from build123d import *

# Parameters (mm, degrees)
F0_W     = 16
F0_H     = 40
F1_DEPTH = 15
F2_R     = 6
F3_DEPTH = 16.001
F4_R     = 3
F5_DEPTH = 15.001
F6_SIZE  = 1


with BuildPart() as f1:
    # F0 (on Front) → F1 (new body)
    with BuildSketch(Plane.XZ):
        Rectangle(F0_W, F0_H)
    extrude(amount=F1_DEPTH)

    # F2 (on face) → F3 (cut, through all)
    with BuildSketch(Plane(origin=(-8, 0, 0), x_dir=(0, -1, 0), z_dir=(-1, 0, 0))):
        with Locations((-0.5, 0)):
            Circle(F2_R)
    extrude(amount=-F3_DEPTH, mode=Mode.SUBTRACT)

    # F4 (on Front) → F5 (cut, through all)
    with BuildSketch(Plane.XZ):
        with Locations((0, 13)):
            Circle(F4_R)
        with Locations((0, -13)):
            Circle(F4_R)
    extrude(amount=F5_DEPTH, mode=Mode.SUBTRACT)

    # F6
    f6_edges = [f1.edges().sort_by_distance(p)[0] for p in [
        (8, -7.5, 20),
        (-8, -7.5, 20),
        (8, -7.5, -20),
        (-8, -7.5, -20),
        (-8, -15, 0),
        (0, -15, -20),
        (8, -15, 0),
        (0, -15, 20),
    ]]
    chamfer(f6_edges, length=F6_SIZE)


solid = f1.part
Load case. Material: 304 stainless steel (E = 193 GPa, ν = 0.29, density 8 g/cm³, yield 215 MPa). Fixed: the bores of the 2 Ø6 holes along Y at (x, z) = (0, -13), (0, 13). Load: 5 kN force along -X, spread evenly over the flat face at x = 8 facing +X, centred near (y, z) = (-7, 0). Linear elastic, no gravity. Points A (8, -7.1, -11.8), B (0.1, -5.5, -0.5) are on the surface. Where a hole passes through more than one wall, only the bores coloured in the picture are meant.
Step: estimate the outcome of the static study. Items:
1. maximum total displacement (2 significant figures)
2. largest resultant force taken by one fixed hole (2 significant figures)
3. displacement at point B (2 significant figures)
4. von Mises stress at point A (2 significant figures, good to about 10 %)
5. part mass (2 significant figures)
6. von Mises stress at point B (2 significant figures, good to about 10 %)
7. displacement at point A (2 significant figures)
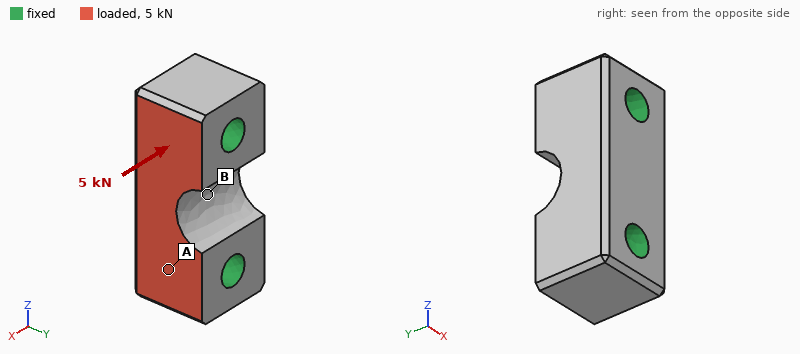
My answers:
0.96 µm
2.5 kN
0.68 µm
14 MPa
63 g
5.3 MPa
0.39 µm
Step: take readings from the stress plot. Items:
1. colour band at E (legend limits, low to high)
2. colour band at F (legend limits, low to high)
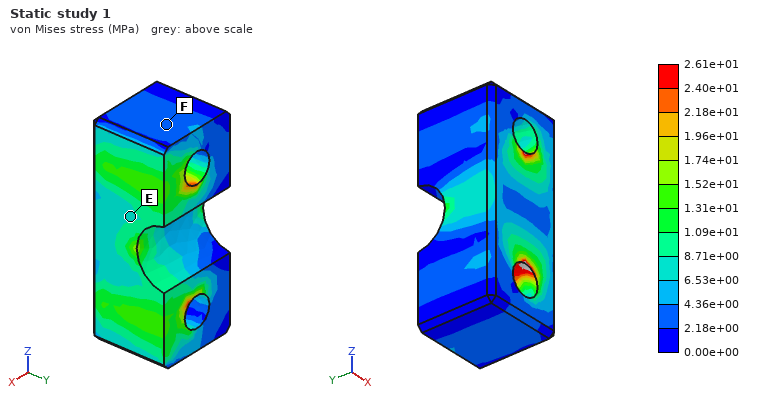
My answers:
6.53e+00 to 8.71e+00 MPa
2.18e+00 to 4.36e+00 MPa
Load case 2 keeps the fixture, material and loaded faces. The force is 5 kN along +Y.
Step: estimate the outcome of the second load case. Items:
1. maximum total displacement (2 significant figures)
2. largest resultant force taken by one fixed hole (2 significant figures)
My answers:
2.7 µm
2.5 kN
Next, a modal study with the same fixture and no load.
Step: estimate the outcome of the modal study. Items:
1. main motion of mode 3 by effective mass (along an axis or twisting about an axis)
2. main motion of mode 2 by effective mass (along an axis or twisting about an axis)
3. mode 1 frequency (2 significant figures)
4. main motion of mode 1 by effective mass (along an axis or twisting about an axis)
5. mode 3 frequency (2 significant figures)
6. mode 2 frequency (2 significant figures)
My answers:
twisting about Z
along Y
53 kHz
along X
69 kHz
59 kHz
